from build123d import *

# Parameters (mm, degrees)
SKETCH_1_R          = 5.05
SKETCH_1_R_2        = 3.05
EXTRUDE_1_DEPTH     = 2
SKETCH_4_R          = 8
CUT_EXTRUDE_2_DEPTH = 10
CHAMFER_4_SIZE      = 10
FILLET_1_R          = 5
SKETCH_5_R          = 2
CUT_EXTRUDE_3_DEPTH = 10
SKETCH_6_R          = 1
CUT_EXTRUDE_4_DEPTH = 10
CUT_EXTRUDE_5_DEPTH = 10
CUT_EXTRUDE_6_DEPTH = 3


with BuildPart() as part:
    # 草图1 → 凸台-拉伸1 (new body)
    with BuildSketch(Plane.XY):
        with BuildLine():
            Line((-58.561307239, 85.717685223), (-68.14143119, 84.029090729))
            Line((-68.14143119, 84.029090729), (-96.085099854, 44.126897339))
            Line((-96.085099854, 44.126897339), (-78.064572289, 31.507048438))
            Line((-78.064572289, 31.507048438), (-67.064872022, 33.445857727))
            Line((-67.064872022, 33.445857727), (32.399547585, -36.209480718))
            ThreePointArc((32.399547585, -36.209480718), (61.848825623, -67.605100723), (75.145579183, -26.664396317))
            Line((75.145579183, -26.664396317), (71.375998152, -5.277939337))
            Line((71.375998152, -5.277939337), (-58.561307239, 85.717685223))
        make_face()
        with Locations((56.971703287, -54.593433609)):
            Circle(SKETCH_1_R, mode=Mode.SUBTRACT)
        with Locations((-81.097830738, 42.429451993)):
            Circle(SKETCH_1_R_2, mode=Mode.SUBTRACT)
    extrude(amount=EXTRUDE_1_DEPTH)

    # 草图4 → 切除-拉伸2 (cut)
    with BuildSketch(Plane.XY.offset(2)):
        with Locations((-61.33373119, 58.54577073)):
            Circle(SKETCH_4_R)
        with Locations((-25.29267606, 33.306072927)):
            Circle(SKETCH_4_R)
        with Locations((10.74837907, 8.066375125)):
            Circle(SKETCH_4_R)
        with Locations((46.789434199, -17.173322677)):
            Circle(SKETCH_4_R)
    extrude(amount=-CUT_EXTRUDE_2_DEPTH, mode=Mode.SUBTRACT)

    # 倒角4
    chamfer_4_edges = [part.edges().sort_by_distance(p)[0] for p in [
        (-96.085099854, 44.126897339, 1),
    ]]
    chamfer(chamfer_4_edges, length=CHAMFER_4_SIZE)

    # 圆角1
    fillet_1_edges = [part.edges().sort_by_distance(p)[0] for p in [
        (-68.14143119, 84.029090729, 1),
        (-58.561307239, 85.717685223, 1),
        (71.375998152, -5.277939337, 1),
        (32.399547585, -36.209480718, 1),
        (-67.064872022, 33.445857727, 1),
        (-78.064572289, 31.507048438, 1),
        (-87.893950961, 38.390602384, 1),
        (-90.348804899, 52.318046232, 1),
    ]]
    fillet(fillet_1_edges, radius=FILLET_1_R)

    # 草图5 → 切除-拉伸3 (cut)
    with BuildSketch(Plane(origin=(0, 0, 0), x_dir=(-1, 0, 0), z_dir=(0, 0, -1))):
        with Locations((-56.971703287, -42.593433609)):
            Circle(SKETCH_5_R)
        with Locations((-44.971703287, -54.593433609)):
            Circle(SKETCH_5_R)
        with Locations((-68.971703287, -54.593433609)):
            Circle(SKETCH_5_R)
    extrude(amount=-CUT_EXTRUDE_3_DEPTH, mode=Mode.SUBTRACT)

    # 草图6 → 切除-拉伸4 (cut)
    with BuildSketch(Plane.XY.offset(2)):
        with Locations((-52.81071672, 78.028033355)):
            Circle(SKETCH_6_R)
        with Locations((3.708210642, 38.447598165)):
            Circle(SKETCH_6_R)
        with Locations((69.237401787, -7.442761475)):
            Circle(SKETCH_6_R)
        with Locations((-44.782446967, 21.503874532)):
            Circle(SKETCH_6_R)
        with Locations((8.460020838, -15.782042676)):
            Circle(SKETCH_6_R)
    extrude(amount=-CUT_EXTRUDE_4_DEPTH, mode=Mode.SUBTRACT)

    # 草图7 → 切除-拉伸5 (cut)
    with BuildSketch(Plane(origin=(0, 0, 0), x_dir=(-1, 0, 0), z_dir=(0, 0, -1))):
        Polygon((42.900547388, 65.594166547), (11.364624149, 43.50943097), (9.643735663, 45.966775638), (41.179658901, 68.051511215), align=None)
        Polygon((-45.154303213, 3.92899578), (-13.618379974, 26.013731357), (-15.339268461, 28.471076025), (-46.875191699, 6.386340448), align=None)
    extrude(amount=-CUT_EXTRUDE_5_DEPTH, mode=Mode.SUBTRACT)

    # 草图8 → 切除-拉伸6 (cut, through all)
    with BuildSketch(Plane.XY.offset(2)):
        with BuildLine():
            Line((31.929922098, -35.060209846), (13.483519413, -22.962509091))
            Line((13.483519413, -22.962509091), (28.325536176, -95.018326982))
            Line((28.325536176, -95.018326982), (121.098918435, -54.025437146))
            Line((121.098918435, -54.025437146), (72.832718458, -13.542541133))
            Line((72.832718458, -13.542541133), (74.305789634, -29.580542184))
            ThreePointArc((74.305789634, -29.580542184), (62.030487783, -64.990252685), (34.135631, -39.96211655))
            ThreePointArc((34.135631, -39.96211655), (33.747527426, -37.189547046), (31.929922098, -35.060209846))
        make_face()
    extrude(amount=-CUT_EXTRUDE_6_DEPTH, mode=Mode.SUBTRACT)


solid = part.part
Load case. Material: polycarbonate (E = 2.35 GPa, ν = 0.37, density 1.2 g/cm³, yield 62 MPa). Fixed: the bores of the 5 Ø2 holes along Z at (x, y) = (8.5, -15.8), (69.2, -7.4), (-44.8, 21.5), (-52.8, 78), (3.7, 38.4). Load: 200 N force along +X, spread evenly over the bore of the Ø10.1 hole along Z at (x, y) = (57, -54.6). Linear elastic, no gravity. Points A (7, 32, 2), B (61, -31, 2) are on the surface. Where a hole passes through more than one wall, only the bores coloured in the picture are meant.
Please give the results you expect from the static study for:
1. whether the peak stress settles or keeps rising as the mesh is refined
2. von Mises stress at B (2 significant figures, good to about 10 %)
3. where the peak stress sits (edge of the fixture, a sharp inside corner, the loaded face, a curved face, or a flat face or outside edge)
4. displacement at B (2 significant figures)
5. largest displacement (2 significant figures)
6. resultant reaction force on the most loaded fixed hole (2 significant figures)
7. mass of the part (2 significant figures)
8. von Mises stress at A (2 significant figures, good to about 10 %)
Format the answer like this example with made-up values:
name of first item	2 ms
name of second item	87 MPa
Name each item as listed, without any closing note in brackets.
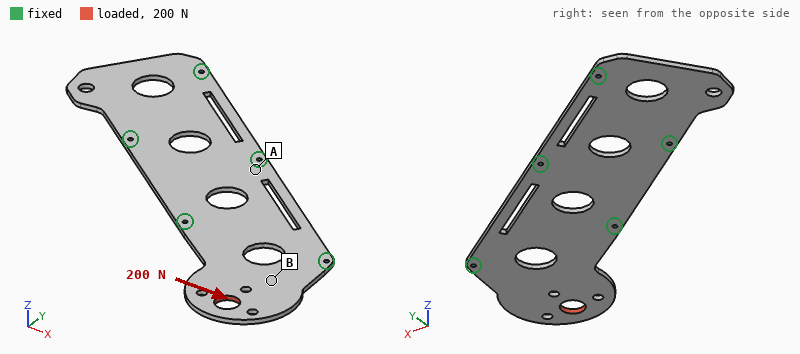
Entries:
whether the peak stress settles or keeps rising as the mesh is refined	keeps rising
von Mises stress at B	3.7 MPa
where the peak stress sits	edge of the fixture
displacement at B	0.12 mm
largest displacement	0.41 mm
resultant reaction force on the most loaded fixed hole	160 N
mass of the part	20 g
von Mises stress at A	1.6 MPa
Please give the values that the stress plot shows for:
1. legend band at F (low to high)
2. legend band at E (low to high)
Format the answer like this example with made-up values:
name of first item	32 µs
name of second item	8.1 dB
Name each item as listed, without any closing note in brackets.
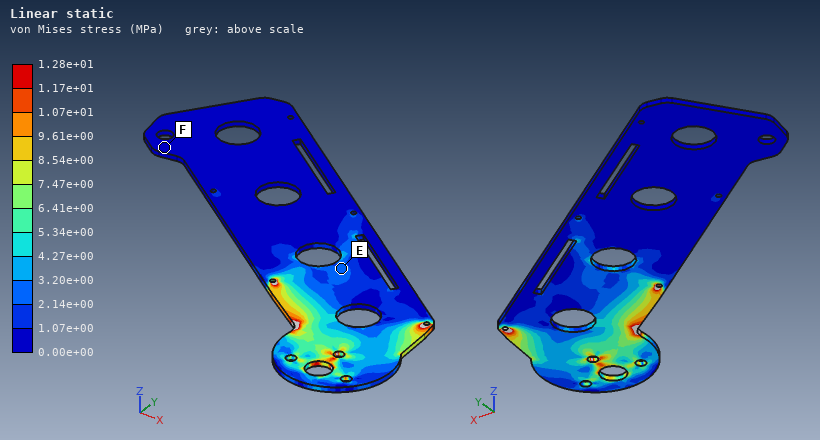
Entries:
legend band at F	0.00e+00 to 1.07e+00 MPa
legend band at E	2.14e+00 to 3.20e+00 MPa
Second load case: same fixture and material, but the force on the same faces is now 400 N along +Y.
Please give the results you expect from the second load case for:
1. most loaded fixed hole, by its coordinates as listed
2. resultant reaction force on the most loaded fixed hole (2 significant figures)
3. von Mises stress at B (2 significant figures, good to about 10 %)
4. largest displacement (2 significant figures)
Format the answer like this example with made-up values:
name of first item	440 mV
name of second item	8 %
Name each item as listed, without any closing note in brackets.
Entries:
most loaded fixed hole, by its coordinates as listed	(69.2, -7.4)
resultant reaction force on the most loaded fixed hole	300 N
von Mises stress at B	6.6 MPa
largest displacement	0.25 mm
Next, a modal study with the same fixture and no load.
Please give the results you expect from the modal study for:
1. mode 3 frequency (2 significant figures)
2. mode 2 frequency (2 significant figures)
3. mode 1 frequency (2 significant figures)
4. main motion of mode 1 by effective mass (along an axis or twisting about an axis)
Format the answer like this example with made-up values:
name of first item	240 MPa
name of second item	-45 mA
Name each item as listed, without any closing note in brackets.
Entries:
mode 3 frequency	460 Hz
mode 2 frequency	270 Hz
mode 1 frequency	140 Hz
main motion of mode 1 by effective mass	along Z
